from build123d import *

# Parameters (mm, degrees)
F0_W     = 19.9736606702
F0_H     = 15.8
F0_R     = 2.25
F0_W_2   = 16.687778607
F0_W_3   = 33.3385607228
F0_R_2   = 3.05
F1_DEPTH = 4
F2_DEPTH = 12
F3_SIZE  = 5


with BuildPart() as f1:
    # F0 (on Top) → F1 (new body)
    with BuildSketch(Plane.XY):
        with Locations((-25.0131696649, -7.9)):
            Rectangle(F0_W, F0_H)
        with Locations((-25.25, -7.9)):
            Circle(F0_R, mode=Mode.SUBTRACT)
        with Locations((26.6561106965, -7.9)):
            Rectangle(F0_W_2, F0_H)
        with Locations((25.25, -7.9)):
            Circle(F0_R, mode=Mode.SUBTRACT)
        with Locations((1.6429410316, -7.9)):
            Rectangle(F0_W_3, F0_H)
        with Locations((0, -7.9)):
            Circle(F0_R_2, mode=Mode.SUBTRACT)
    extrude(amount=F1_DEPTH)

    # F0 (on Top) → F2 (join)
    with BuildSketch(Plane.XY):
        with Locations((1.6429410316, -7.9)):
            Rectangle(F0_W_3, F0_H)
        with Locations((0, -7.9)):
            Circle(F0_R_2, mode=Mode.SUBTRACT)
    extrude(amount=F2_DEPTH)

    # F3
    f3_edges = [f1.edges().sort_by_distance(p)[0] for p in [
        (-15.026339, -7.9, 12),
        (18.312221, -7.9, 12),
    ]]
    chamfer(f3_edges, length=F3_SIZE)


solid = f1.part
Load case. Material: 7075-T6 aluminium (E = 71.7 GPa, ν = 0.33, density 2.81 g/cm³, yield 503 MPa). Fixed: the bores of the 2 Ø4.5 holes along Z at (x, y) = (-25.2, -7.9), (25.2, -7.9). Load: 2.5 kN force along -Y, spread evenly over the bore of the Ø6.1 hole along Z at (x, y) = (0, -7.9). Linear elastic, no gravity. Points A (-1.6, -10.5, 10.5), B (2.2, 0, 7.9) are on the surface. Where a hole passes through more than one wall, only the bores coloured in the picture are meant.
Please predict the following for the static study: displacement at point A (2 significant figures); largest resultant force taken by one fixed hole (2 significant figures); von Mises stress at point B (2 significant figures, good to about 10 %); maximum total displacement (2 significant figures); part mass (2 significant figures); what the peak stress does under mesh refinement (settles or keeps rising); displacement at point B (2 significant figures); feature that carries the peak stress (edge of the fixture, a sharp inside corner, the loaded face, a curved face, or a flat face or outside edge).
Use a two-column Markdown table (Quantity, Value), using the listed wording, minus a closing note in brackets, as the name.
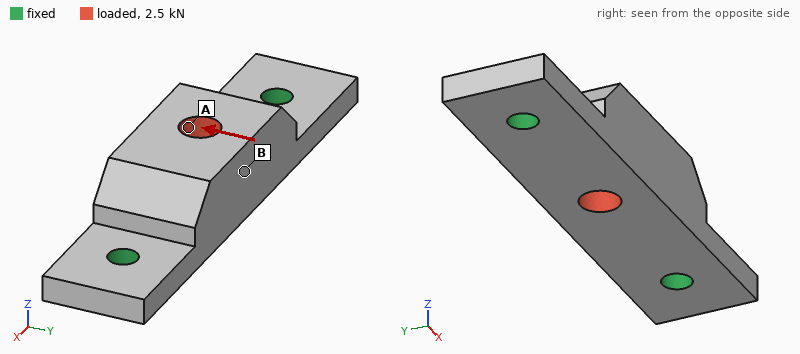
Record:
| Quantity | Value |
|---|---|
| displacement at point A | 67 µm |
| largest resultant force taken by one fixed hole | 1.3 kN |
| von Mises stress at point B | 43 MPa |
| maximum total displacement | 81 µm |
| part mass | 22 g |
| what the peak stress does under mesh refinement | keeps rising |
| displacement at point B | 64 µm |
| feature that carries the peak stress | edge of the fixture |
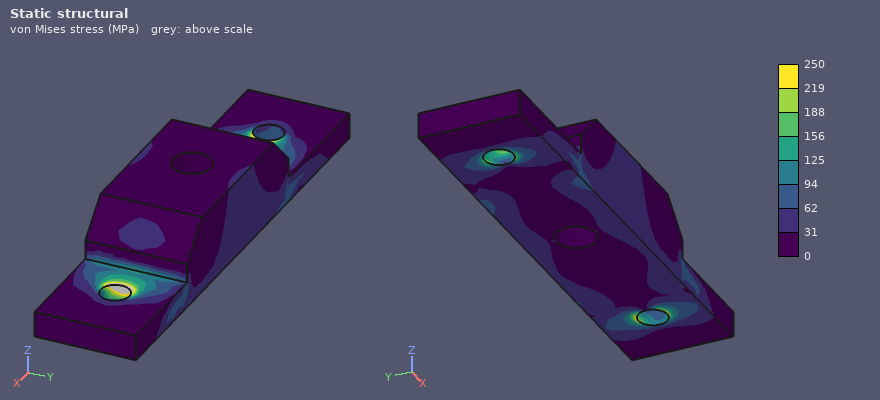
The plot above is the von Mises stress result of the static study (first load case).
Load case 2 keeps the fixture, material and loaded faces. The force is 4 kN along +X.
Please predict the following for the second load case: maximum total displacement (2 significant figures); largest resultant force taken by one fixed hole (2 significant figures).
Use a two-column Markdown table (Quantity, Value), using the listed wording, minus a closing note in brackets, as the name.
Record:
| Quantity | Value |
|---|---|
| maximum total displacement | 12 µm |
| largest resultant force taken by one fixed hole | 2.1 kN |
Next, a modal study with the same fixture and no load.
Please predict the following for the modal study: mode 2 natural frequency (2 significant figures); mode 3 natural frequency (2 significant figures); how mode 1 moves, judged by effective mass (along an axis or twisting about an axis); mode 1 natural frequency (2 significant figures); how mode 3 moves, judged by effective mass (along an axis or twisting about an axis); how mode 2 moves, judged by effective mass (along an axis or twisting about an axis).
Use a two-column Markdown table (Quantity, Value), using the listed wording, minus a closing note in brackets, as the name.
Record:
| Quantity | Value |
|---|---|
| mode 2 natural frequency | 10 kHz |
| mode 3 natural frequency | 17 kHz |
| how mode 1 moves, judged by effective mass | along Y |
| mode 1 natural frequency | 8200 Hz |
| how mode 3 moves, judged by effective mass | along Y |
| how mode 2 moves, judged by effective mass | along Z |
